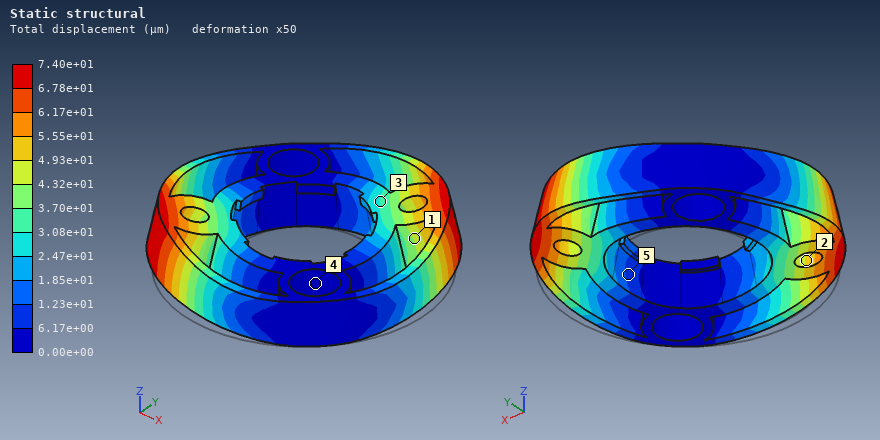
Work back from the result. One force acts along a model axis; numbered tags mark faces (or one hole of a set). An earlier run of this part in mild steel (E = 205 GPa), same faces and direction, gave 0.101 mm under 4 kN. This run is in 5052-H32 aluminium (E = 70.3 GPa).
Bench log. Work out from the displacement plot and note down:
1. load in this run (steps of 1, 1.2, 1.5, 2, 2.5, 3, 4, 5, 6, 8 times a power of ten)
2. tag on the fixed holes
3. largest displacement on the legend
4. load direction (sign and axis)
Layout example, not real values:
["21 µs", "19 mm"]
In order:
["1 kN", "4", "7.40e+01 µm", "+Z"]
